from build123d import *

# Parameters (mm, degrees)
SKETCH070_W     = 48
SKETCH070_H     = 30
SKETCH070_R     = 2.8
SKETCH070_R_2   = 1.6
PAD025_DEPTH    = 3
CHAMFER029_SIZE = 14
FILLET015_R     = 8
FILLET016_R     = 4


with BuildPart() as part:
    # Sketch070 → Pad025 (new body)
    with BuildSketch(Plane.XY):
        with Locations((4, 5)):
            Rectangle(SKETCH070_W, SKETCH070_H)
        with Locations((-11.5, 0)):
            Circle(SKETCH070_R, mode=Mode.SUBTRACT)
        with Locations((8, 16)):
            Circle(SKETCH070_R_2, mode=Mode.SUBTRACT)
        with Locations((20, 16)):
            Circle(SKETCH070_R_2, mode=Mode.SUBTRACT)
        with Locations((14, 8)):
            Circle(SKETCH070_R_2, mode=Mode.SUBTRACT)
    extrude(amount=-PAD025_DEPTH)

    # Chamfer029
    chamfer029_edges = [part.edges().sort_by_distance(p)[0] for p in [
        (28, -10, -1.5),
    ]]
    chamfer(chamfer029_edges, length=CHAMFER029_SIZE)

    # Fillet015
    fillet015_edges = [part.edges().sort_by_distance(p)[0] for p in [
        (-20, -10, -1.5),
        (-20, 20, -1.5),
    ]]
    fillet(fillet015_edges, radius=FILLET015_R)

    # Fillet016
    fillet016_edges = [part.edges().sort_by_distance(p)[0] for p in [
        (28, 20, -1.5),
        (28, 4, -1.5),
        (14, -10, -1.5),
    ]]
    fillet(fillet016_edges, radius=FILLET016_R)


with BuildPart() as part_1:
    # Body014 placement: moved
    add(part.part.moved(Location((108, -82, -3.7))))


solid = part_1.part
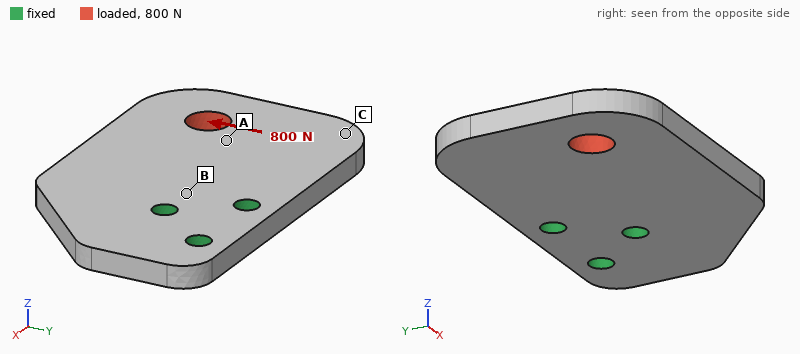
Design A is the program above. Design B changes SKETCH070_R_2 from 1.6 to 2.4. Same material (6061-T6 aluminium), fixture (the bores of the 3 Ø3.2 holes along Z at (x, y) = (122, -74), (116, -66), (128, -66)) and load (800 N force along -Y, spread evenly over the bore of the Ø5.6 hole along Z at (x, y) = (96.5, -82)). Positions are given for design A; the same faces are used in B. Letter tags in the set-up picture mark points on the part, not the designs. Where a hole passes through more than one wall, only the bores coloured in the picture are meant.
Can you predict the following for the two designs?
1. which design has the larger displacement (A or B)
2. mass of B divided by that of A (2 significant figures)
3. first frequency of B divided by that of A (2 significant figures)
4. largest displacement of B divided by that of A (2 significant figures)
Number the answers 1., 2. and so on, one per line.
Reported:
1. A
2. 0.98
3. 1.1
4. 0.84
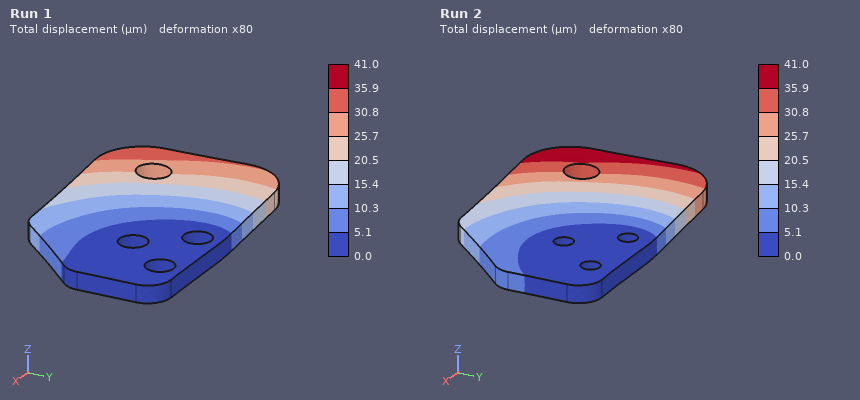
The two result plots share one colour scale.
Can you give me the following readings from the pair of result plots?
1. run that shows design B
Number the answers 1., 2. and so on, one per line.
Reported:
1. Run 1
